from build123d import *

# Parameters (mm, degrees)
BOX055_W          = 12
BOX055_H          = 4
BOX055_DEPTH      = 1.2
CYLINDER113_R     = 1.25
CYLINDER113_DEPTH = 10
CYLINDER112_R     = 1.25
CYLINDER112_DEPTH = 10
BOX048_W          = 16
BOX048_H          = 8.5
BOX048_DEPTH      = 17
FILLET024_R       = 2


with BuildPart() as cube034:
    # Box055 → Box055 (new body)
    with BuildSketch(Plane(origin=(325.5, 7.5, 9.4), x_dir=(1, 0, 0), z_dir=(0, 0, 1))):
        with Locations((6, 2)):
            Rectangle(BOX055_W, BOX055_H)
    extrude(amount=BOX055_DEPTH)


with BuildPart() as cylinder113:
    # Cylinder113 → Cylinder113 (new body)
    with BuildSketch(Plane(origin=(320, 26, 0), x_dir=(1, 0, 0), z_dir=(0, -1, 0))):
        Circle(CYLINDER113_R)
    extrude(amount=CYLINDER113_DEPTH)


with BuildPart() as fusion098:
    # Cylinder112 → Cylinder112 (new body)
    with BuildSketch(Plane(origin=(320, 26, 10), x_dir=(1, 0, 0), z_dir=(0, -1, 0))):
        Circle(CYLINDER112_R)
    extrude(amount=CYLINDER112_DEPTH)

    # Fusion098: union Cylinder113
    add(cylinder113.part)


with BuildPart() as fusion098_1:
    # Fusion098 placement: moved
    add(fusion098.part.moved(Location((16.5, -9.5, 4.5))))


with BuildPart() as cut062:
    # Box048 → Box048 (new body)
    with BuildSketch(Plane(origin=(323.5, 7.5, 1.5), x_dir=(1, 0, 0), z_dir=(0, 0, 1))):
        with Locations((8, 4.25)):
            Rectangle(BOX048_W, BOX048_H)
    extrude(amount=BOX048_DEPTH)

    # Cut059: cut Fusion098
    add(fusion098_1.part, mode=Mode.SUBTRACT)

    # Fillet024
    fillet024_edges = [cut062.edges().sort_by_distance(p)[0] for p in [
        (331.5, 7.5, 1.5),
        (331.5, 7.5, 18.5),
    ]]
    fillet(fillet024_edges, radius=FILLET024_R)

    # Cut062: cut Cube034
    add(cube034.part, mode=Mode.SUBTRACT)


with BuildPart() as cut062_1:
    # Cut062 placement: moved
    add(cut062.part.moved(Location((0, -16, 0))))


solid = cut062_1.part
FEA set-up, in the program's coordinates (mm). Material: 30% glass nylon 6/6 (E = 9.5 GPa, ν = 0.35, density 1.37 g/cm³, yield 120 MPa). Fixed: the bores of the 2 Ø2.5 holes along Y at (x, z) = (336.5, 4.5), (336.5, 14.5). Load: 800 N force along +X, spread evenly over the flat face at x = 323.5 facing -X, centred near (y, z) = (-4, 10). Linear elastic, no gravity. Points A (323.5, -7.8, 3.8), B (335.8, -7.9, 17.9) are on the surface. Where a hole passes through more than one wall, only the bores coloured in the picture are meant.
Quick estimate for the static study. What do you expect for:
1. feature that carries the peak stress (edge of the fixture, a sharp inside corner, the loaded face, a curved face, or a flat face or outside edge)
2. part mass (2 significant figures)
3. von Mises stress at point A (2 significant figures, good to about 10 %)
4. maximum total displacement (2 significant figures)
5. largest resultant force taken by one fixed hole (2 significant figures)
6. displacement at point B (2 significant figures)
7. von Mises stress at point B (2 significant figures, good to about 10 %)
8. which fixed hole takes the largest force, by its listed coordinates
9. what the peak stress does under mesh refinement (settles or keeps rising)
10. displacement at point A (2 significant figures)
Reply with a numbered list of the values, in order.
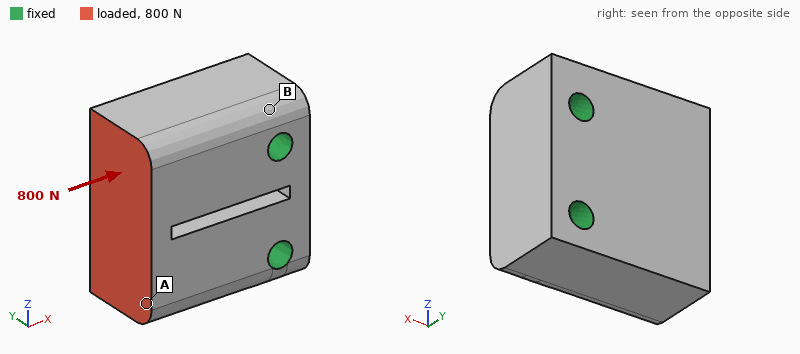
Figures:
1. edge of the fixture
2. 2.9 g
3. 5.6 MPa
4. 9.4 µm
5. 430 N
6. 2.3 µm
7. 3.3 MPa
8. (336.5, 14.5)
9. keeps rising
10. 8.3 µm
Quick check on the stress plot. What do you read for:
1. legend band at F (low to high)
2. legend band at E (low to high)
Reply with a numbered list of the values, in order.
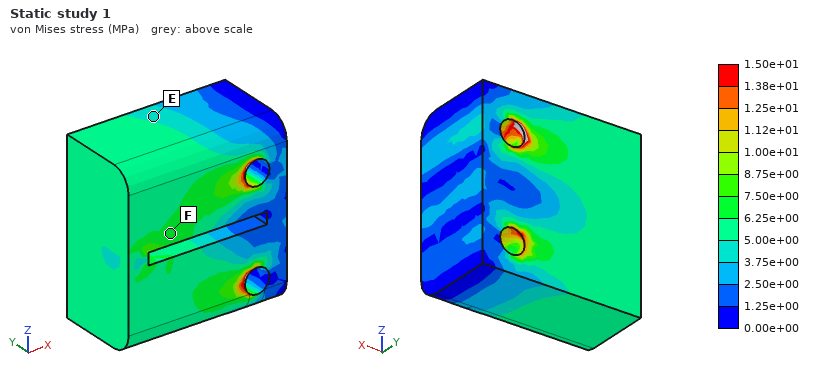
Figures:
1. 6.25e+00 to 7.50e+00 MPa
2. 3.75e+00 to 5.00e+00 MPa
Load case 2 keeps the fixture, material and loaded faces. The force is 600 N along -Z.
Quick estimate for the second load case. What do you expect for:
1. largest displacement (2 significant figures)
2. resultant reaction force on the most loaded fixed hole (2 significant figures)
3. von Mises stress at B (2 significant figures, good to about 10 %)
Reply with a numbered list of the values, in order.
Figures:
1. 50 µm
2. 690 N
3. 11 MPa
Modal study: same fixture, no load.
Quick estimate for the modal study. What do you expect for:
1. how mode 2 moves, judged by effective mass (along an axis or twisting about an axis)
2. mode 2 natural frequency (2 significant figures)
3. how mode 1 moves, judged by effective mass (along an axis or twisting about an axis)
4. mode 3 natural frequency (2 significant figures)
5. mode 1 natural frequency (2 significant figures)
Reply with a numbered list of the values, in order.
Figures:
1. along Z
2. 20 kHz
3. along Y
4. 25 kHz
5. 16 kHz
